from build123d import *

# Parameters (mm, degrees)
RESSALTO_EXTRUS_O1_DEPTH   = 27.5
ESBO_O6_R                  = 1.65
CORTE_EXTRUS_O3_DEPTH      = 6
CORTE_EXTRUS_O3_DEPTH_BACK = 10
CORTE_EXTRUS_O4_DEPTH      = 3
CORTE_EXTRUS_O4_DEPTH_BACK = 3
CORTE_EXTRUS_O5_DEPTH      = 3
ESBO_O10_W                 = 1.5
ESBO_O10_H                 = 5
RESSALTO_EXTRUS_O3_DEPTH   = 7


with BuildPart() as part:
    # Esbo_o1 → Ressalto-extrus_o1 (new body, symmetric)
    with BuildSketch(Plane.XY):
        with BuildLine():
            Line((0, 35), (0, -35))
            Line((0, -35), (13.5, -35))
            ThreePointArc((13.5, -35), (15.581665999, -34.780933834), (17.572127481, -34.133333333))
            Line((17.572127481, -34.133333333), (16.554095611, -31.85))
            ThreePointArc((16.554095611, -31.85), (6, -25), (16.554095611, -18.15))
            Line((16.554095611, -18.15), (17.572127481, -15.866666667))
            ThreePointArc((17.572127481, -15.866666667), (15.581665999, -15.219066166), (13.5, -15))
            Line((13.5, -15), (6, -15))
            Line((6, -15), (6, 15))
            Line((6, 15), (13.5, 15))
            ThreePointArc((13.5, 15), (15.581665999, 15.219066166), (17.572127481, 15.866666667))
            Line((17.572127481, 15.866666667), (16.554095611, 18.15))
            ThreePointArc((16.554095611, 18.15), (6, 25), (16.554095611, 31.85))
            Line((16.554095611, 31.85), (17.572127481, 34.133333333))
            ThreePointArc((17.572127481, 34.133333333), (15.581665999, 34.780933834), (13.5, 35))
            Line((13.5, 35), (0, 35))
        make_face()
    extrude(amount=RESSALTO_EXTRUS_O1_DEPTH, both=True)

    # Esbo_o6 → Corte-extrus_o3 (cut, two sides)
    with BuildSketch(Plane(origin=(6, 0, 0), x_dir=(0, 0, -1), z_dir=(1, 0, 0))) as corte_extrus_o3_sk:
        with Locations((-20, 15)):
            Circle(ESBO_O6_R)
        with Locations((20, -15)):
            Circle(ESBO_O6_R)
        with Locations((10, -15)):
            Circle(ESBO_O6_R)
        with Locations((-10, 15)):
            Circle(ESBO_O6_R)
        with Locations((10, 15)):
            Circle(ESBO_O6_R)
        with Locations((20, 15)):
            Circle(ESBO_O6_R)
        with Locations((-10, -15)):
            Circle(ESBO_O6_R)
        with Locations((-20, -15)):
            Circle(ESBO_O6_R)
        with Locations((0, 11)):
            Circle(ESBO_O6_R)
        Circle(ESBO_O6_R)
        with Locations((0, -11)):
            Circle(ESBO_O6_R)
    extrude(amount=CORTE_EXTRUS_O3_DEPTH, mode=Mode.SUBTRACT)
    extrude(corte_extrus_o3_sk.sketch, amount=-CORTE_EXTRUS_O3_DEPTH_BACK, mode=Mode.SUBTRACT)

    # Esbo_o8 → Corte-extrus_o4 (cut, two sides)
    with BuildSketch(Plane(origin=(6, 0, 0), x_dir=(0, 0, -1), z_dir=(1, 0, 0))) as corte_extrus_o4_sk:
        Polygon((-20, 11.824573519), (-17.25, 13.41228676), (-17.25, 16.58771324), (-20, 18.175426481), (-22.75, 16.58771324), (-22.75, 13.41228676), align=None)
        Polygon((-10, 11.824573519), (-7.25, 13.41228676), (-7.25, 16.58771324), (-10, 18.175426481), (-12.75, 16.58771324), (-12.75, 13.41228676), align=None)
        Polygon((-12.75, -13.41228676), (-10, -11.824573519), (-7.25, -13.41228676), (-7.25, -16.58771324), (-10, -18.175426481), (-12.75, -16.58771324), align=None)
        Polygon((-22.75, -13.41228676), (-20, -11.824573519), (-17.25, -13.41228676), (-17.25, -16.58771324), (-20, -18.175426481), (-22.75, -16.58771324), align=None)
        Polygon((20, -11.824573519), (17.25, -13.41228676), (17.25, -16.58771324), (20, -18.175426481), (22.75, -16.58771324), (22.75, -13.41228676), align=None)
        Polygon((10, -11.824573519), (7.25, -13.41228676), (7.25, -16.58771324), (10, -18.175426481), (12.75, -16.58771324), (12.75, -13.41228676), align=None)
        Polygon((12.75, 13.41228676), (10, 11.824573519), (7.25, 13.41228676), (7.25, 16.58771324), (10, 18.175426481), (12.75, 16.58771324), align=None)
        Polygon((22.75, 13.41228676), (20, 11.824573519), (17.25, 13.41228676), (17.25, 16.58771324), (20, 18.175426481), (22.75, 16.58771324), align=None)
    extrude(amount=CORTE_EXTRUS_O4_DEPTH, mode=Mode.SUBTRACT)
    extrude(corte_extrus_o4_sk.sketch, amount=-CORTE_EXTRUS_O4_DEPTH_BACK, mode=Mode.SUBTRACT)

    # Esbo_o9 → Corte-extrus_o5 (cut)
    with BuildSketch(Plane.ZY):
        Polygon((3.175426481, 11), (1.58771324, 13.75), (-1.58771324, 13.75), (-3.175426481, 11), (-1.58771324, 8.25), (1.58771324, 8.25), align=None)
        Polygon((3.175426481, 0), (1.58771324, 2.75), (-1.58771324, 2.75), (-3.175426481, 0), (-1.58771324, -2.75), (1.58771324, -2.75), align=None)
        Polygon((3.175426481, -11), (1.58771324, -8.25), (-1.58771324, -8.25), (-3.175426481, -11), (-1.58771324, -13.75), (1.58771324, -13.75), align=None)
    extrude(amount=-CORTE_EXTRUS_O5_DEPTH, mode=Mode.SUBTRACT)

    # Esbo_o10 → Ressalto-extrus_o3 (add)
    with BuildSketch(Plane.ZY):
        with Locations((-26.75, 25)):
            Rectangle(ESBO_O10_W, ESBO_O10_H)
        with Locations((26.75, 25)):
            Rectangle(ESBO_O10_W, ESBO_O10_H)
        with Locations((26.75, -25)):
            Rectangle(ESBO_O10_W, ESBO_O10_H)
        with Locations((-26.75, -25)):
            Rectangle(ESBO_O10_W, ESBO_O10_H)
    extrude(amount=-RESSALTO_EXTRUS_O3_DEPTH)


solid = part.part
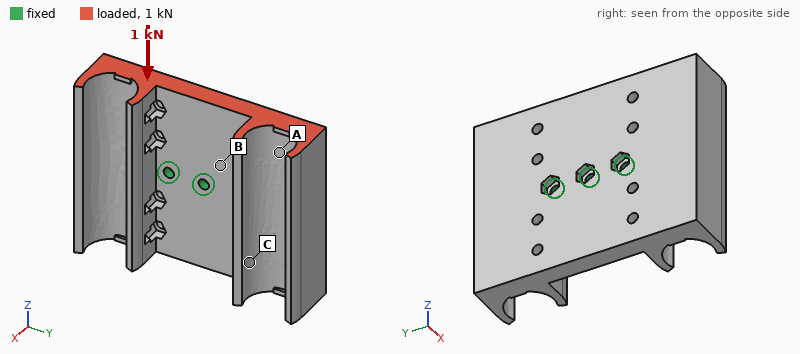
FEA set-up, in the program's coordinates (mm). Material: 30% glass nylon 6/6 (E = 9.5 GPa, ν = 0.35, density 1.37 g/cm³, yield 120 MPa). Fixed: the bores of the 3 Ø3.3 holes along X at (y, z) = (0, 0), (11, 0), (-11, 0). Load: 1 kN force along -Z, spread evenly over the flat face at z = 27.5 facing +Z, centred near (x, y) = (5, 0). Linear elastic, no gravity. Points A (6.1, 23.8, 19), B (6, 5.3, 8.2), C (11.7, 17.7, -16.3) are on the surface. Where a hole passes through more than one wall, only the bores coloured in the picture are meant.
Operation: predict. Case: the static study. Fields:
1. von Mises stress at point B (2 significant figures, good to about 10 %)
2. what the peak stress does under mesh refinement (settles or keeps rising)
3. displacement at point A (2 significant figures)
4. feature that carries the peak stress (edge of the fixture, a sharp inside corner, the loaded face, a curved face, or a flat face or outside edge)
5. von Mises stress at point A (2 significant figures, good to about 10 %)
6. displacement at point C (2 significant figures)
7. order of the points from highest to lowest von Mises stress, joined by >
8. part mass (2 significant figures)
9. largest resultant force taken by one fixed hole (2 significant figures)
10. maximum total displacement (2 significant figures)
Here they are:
4.3 MPa
keeps rising
28 µm
edge of the fixture
2.5 MPa
24 µm
B > A > C
42 g
380 N
54 µm
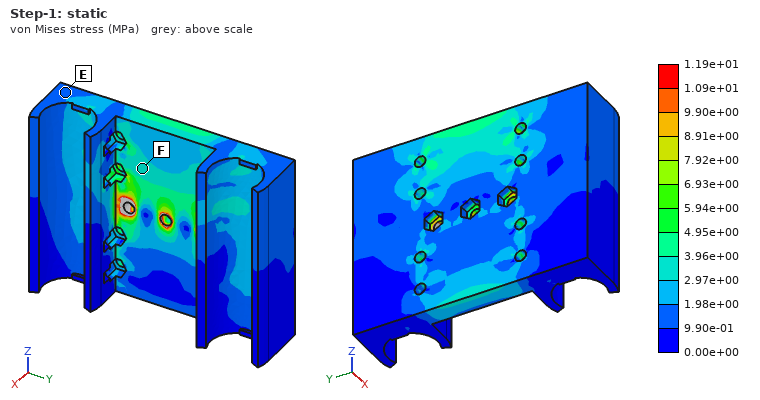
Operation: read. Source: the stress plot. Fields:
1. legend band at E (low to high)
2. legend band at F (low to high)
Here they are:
9.90e-01 to 1.98e+00 MPa
2.97e+00 to 3.96e+00 MPa
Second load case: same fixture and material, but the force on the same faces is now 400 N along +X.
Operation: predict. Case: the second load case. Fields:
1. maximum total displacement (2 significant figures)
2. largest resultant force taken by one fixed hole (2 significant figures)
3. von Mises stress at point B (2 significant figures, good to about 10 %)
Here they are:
0.65 mm
250 N
14 MPa
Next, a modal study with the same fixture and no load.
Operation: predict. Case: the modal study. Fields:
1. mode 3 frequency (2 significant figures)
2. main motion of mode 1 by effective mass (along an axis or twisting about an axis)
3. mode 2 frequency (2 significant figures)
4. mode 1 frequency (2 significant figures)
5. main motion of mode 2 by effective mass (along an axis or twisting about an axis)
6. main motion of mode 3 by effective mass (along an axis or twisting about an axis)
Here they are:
2000 Hz
twisting about Y
1800 Hz
1200 Hz
twisting about Z
along X
